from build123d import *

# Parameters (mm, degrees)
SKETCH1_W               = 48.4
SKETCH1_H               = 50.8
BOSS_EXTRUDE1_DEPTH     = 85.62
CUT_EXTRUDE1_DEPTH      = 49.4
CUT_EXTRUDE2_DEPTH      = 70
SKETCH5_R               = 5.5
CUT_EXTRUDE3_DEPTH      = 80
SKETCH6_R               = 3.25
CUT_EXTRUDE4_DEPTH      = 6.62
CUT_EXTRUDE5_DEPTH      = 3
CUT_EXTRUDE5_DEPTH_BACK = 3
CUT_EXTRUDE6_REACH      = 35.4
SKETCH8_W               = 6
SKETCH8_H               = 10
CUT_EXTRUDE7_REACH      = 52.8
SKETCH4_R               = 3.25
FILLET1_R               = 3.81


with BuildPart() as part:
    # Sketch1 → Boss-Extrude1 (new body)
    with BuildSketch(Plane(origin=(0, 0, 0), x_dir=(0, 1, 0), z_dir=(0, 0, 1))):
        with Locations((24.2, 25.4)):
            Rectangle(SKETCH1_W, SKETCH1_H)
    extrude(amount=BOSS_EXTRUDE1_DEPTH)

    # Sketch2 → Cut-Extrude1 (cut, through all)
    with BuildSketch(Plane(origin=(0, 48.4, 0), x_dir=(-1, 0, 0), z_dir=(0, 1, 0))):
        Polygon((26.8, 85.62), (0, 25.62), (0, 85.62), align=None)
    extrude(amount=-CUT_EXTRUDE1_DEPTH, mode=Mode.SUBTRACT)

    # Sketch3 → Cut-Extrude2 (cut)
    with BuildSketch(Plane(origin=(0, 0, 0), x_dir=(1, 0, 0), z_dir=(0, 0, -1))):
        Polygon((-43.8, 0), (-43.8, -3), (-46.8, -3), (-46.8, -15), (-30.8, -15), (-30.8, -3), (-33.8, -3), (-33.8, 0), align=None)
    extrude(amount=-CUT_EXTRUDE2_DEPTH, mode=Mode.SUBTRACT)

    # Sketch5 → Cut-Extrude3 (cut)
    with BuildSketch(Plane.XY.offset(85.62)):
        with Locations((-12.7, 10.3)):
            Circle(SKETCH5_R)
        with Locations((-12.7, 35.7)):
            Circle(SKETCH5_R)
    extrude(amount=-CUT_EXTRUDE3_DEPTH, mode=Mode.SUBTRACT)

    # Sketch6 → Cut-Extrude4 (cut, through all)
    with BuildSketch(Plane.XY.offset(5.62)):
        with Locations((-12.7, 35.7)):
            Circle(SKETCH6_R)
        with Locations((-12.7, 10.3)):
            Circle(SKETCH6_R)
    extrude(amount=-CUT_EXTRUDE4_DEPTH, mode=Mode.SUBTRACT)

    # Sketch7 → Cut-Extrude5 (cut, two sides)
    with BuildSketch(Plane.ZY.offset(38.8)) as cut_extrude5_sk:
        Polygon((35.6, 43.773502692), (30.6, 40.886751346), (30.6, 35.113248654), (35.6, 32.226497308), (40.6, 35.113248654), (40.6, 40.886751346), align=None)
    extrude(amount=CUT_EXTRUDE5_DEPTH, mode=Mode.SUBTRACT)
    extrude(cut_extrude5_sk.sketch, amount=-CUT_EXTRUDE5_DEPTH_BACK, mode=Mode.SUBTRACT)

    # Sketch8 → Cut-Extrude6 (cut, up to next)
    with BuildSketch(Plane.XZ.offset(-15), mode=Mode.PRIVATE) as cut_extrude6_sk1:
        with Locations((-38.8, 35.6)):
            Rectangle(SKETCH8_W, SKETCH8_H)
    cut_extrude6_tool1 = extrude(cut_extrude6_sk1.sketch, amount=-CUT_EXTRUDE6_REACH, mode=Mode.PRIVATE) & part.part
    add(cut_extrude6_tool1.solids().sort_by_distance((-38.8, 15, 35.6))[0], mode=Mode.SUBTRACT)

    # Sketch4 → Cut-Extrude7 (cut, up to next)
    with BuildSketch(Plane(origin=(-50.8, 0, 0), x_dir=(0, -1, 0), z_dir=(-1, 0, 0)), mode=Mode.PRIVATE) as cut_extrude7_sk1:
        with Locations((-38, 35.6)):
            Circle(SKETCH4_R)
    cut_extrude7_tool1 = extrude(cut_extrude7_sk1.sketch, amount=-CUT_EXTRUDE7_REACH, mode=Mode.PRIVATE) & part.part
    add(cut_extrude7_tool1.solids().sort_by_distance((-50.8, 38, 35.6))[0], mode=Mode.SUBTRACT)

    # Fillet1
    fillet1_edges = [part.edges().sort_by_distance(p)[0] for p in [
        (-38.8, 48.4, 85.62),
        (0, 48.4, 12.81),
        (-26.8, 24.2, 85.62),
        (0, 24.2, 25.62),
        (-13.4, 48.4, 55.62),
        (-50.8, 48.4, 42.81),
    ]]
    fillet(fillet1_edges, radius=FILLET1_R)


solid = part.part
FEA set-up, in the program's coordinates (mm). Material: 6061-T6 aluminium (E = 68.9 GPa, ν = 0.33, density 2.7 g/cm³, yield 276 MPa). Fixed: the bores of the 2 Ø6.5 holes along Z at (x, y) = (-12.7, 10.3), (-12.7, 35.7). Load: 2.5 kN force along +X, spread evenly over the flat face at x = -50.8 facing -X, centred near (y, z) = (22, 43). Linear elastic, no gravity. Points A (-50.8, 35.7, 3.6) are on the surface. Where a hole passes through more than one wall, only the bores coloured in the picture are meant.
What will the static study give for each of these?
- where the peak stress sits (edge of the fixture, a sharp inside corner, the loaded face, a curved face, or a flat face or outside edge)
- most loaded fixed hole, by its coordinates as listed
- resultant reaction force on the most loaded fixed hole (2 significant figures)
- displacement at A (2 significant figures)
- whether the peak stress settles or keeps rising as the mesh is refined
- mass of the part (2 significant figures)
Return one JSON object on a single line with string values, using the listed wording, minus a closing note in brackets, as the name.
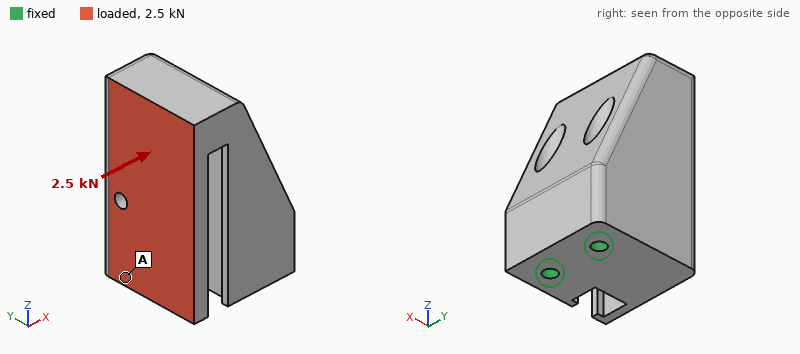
{"where the peak stress sits": "edge of the fixture", "most loaded fixed hole, by its coordinates as listed": "(-12.7, 10.3)", "resultant reaction force on the most loaded fixed hole": "1.3 kN", "displacement at A": "0.14 mm", "whether the peak stress settles or keeps rising as the mesh is refined": "keeps rising", "mass of the part": "390 g"}
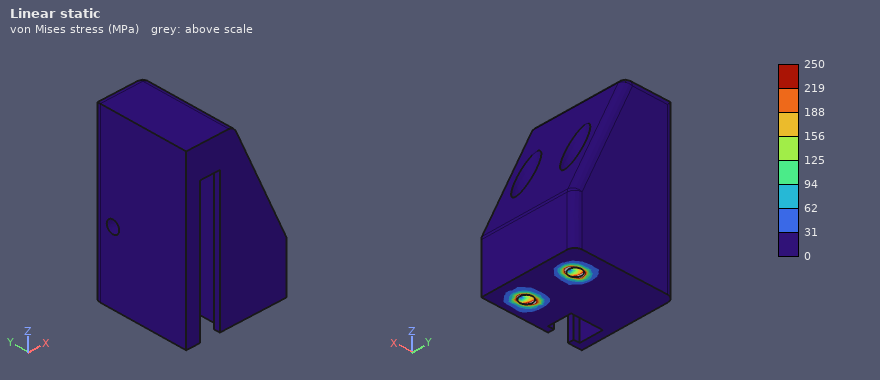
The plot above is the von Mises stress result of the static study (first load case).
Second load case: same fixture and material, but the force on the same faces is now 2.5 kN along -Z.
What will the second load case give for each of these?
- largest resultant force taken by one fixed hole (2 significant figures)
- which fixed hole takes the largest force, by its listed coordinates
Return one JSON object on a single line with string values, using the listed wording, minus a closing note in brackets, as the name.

{"largest resultant force taken by one fixed hole": "1.3 kN", "which fixed hole takes the largest force, by its listed coordinates": "(-12.7, 10.3)"}
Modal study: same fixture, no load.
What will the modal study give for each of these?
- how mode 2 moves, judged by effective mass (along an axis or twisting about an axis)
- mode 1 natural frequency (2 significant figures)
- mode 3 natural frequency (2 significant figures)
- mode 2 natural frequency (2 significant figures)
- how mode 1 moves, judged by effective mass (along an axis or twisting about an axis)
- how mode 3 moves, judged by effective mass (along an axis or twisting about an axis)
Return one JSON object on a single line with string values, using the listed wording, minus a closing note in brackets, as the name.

{"how mode 2 moves, judged by effective mass": "along Y", "mode 1 natural frequency": "880 Hz", "mode 3 natural frequency": "5600 Hz", "mode 2 natural frequency": "2300 Hz", "how mode 1 moves, judged by effective mass": "along X", "how mode 3 moves, judged by effective mass": "twisting about Z"}
